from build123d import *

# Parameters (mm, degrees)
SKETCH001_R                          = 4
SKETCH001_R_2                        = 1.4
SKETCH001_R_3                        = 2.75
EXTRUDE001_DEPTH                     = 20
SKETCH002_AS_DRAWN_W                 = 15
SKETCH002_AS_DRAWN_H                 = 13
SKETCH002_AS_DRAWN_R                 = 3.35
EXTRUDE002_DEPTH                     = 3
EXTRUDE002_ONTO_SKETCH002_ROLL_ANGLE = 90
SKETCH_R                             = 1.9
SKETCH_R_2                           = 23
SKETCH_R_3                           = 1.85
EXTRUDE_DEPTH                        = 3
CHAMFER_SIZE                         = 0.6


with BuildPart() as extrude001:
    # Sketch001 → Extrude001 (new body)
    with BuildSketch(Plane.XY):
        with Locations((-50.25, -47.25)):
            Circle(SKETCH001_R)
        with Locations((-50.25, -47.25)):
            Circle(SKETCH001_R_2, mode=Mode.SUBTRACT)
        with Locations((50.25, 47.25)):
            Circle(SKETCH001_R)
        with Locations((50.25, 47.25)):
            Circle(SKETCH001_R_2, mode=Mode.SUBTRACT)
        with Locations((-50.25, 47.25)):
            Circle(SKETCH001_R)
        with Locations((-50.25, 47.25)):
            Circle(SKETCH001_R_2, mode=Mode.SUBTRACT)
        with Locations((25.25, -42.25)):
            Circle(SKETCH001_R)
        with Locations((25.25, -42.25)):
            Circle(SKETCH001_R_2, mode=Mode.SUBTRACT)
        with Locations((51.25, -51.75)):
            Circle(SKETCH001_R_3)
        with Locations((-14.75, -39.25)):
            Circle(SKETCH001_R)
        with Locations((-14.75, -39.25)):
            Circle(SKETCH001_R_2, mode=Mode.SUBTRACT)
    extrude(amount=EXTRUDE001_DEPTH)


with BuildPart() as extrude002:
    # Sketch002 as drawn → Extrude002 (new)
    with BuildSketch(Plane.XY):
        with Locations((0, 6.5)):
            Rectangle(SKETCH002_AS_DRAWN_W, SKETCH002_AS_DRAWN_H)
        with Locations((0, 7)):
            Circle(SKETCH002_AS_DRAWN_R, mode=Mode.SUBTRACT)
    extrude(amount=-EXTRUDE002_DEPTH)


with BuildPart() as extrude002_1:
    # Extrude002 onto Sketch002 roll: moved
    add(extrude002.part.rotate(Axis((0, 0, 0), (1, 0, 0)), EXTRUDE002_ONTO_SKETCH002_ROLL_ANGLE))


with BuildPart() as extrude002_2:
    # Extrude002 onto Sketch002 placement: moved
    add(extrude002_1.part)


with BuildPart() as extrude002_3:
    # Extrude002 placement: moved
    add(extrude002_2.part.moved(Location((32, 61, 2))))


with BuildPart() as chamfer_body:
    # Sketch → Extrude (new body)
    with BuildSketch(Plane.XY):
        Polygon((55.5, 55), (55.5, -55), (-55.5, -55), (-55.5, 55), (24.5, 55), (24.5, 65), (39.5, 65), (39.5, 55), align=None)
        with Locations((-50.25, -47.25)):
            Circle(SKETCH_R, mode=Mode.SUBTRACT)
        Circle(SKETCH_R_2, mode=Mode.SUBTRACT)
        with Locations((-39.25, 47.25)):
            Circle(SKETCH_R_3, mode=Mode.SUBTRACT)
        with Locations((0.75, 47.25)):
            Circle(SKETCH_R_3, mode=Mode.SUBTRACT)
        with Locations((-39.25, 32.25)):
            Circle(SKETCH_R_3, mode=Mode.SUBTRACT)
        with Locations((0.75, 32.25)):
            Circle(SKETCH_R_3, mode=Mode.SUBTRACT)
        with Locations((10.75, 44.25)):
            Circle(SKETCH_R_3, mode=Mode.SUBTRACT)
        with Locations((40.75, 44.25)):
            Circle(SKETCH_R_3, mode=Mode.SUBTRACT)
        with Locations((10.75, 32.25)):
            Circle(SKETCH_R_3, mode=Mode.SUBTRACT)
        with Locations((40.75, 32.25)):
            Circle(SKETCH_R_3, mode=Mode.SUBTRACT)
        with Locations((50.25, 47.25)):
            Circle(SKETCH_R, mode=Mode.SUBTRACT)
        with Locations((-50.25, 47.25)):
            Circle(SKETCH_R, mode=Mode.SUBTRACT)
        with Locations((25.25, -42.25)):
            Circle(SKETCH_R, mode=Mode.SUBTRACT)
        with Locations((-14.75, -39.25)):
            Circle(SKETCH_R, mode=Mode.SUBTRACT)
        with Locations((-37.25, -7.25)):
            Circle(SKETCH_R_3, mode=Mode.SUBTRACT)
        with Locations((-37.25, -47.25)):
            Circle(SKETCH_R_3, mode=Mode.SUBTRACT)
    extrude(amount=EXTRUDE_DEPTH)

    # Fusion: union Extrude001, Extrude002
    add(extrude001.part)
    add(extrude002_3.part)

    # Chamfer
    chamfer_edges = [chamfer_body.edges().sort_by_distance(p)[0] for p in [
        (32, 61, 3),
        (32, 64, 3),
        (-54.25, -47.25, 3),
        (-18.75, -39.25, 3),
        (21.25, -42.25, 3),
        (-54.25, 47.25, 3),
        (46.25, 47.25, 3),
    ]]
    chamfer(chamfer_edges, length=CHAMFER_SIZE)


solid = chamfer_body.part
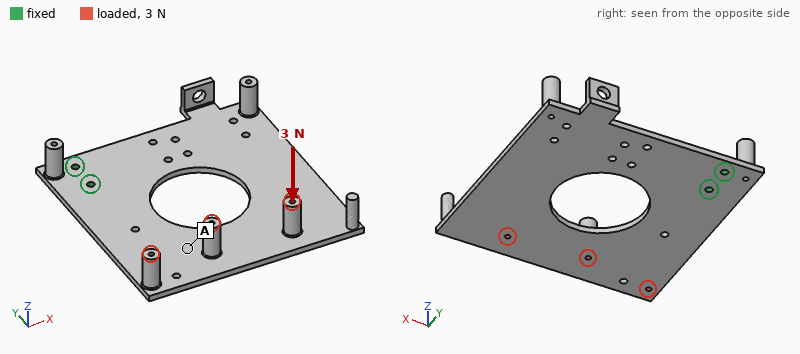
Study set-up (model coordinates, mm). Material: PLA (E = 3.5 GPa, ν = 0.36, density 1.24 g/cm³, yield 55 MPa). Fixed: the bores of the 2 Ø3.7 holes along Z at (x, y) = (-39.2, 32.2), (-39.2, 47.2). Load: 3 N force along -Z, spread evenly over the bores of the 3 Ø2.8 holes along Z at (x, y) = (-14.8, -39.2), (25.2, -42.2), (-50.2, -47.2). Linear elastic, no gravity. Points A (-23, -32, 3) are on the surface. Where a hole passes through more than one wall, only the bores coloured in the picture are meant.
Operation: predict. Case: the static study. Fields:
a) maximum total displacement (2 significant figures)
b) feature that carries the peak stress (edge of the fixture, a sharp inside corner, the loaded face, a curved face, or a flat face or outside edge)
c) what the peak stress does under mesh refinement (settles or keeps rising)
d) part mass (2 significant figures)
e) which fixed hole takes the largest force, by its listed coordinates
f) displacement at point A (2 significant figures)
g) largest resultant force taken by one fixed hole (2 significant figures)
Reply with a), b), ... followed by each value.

a) 1.9 mm
b) edge of the fixture
c) keeps rising
d) 45 g
e) (-39.2, 32.2)
f) 0.93 mm
g) 11 N
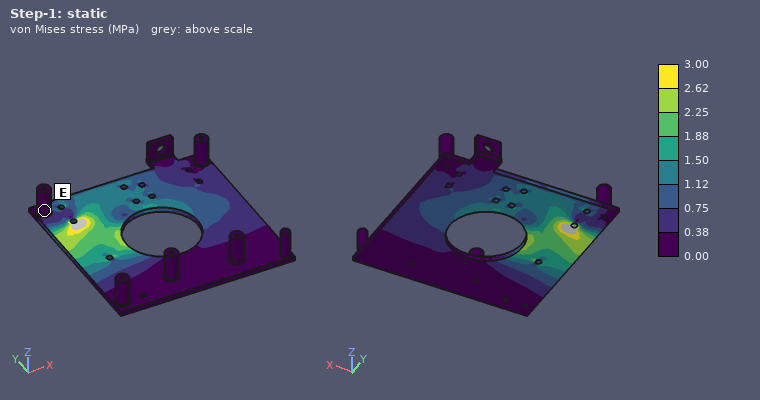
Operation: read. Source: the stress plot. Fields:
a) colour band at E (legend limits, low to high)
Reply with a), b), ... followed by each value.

a) 0.00 to 0.38 MPa
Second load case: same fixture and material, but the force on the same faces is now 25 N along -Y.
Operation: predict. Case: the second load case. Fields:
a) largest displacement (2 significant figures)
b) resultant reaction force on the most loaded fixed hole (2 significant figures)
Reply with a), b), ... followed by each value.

a) 2.0 mm
b) 42 N
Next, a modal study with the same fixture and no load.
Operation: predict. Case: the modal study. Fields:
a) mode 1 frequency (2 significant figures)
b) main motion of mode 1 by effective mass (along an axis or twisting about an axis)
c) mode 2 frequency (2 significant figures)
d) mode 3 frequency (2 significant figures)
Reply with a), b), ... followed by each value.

a) 48 Hz
b) along Z
c) 81 Hz
d) 170 Hz
